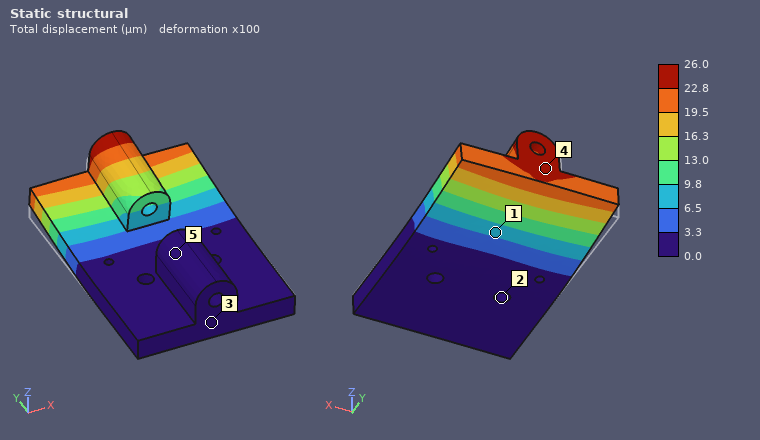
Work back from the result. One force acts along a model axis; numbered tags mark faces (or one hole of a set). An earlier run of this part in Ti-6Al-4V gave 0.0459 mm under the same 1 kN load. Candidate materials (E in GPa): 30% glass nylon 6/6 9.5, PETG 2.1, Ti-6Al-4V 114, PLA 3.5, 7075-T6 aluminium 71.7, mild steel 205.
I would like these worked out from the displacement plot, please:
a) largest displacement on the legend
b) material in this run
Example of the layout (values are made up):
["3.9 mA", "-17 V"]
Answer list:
["26.0 µm", "mild steel"]
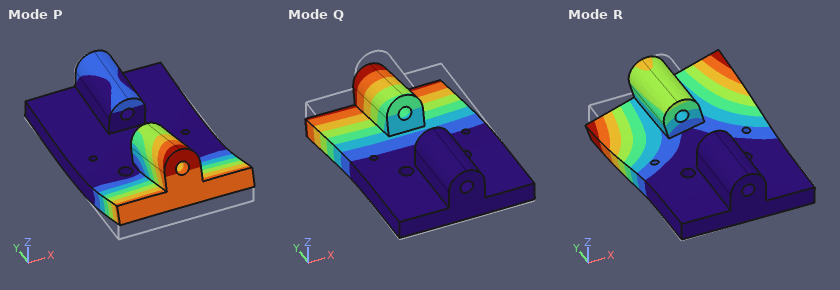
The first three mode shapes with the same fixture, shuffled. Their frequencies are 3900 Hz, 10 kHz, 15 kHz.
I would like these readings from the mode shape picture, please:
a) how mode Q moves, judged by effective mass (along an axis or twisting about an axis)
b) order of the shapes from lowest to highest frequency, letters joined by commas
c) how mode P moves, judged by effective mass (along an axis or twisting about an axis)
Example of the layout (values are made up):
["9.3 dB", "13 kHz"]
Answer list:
["along Z", "Q, R, P", "along Z"]
